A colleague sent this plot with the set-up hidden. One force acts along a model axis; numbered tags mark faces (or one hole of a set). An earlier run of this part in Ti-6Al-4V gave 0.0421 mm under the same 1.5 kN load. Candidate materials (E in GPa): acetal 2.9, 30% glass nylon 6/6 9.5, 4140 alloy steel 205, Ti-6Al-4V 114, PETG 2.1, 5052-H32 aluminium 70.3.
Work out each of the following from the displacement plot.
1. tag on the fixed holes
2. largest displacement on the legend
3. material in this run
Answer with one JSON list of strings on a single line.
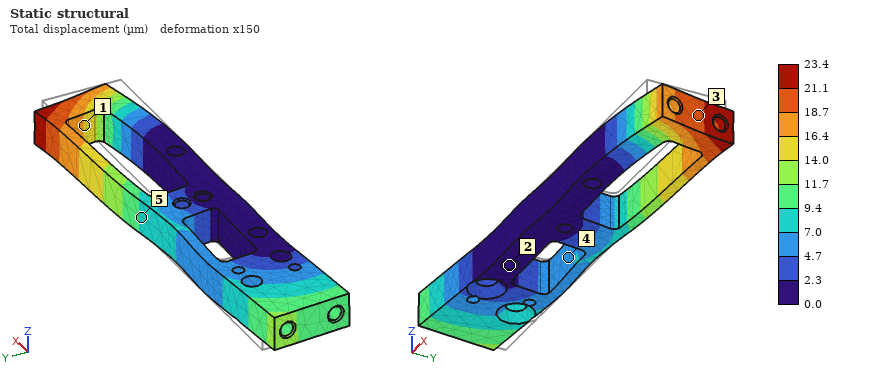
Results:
["2", "23.4 µm", "4140 alloy steel"]
